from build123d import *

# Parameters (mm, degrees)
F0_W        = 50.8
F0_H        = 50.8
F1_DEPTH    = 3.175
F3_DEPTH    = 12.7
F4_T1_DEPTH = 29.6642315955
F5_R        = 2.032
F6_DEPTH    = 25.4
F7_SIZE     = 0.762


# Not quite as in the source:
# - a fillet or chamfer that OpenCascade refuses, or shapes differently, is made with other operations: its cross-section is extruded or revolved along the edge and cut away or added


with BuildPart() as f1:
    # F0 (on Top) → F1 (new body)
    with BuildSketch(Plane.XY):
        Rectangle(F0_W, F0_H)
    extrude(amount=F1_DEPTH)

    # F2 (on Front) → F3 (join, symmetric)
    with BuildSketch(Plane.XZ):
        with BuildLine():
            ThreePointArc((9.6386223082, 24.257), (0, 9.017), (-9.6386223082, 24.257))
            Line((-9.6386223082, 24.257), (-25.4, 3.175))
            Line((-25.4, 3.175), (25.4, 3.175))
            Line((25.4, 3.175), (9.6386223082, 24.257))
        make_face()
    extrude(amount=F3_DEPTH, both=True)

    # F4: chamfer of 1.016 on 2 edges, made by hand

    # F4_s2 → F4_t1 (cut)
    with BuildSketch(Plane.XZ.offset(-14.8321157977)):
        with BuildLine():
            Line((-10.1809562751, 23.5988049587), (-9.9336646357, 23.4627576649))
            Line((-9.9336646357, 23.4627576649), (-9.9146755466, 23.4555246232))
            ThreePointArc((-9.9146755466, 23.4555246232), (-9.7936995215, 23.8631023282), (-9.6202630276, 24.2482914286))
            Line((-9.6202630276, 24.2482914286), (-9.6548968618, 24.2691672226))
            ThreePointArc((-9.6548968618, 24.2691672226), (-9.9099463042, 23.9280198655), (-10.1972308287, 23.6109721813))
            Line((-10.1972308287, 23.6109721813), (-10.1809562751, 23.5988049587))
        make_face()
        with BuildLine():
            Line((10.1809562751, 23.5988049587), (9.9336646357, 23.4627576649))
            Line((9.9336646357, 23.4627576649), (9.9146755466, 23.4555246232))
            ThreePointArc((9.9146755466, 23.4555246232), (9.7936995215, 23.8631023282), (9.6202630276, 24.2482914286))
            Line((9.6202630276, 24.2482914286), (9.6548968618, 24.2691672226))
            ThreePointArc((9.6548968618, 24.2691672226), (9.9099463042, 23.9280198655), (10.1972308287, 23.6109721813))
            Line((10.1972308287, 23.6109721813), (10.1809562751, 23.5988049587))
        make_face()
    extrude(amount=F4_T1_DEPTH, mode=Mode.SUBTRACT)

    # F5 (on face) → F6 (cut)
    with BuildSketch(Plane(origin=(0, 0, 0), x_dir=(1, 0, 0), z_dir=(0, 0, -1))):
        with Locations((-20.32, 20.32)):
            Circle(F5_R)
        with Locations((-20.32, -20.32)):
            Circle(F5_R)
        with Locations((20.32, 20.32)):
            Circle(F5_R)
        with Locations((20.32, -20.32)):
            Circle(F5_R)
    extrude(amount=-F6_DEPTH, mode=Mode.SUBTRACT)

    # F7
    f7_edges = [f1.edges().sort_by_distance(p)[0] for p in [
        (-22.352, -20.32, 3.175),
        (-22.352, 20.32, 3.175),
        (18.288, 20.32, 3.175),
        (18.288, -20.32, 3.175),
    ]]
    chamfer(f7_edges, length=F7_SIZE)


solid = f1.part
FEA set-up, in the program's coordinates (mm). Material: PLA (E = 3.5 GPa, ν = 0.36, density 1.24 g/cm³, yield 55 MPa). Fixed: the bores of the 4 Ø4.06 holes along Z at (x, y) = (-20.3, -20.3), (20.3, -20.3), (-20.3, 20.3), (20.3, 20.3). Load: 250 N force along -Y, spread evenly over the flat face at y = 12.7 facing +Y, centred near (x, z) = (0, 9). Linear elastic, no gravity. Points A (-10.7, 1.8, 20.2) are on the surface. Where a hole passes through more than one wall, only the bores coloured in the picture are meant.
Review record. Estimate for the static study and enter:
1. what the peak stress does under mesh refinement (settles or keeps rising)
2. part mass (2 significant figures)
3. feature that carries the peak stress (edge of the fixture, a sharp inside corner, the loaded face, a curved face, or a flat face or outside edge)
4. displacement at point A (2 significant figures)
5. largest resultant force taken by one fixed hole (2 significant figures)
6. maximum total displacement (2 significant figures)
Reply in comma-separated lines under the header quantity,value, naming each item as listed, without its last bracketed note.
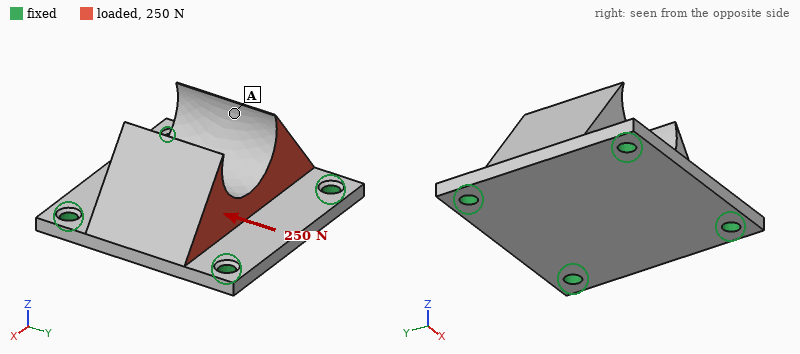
quantity,value
what the peak stress does under mesh refinement,keeps rising
part mass,25 g
feature that carries the peak stress,edge of the fixture
displacement at point A,23 µm
largest resultant force taken by one fixed hole,73 N
maximum total displacement,31 µm
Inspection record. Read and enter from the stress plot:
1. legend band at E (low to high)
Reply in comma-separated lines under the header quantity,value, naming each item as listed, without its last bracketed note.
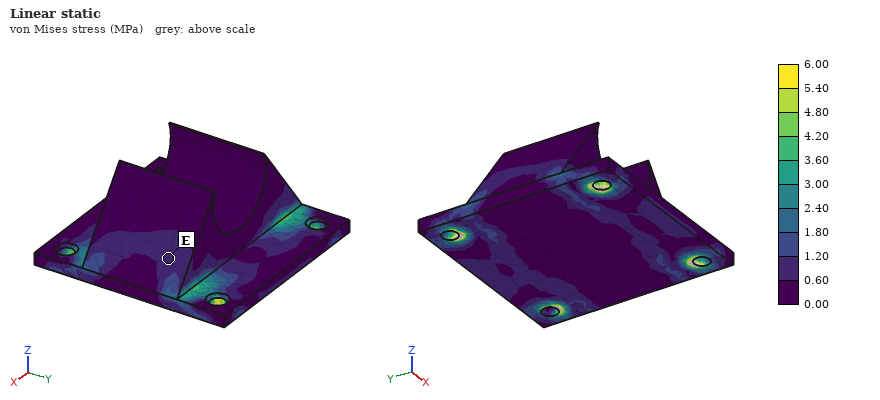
quantity,value
legend band at E,0.60 to 1.20 MPa
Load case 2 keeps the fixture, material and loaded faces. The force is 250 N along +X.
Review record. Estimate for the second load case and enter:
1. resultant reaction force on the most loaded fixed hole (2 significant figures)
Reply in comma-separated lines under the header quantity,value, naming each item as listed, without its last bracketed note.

quantity,value
resultant reaction force on the most loaded fixed hole,87 N
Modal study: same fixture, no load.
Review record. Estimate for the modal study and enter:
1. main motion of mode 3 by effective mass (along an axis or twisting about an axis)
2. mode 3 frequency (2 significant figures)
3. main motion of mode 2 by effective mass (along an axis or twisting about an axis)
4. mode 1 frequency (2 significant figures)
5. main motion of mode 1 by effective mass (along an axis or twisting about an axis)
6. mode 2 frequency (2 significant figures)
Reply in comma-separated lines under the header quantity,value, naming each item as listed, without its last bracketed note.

quantity,value
main motion of mode 3 by effective mass,along Y
mode 3 frequency,3900 Hz
main motion of mode 2 by effective mass,along X
mode 1 frequency,2500 Hz
main motion of mode 1 by effective mass,along Z
mode 2 frequency,3400 Hz
